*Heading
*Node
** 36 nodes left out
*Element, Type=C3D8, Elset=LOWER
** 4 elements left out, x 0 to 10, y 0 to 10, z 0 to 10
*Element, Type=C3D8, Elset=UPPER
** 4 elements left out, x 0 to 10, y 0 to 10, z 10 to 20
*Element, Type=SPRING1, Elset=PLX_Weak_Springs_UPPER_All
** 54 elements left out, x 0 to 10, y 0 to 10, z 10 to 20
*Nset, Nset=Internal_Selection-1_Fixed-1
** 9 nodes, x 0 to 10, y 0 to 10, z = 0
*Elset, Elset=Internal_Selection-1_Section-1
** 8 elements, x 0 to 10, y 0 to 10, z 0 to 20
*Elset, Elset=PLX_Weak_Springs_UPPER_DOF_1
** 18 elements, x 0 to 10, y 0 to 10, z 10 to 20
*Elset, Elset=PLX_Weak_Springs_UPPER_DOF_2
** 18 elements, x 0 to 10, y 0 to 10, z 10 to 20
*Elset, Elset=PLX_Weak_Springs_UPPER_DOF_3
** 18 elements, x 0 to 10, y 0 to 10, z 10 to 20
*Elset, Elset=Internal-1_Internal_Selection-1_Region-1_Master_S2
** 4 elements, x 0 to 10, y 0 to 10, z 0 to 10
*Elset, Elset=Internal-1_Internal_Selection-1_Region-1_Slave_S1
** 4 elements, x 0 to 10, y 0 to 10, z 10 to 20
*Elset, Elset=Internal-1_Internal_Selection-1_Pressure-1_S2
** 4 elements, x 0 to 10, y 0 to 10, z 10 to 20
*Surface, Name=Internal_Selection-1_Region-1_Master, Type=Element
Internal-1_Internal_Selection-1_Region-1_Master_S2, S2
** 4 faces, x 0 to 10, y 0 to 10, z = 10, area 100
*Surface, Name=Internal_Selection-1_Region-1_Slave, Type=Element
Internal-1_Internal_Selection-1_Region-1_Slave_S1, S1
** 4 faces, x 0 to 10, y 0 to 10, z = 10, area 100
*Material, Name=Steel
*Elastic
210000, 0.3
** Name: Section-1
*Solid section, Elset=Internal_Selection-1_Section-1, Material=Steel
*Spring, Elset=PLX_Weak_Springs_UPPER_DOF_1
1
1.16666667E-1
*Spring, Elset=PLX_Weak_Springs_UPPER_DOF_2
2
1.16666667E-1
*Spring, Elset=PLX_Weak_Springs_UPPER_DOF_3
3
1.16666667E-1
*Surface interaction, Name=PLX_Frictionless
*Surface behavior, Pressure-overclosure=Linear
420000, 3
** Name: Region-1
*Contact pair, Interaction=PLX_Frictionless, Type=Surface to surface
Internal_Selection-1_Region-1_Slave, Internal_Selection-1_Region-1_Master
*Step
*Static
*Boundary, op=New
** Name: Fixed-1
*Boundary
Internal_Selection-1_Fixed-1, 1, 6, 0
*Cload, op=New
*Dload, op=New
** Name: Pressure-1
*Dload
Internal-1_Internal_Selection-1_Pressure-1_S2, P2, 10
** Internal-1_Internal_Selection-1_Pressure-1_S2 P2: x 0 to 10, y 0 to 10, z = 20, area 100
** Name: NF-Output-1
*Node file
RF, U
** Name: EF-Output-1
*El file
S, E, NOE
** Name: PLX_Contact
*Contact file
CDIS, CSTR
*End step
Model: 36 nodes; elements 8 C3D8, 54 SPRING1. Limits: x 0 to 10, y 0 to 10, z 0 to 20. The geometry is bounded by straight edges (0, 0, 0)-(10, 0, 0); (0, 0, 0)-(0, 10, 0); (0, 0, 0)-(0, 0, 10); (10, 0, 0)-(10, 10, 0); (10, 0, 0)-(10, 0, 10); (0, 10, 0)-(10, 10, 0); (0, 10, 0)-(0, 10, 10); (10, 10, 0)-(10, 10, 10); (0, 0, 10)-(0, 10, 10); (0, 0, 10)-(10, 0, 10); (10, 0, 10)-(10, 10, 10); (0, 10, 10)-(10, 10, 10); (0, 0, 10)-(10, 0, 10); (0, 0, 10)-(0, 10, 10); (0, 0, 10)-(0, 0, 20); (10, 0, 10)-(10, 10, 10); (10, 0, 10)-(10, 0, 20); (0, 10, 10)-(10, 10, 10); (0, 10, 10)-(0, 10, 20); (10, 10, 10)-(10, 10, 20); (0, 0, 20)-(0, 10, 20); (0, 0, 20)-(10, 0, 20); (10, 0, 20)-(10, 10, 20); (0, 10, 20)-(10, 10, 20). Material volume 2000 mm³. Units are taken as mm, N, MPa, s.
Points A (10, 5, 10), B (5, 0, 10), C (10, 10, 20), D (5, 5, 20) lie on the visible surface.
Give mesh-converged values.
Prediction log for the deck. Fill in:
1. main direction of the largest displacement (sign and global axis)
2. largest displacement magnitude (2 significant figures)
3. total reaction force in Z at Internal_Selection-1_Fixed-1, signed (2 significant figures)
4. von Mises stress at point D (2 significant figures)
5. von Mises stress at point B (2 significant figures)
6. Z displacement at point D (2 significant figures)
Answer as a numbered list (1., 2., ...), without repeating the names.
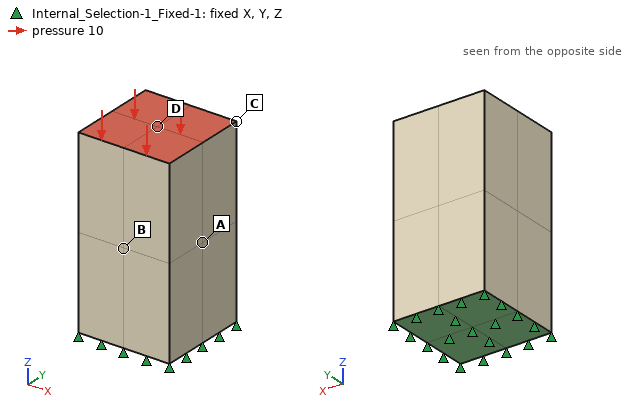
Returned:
1. -Z
2. 9.6e-04 mm
3. 1000 N
4. 10 MPa
5. 11 MPa
6. -9.5e-04 mm
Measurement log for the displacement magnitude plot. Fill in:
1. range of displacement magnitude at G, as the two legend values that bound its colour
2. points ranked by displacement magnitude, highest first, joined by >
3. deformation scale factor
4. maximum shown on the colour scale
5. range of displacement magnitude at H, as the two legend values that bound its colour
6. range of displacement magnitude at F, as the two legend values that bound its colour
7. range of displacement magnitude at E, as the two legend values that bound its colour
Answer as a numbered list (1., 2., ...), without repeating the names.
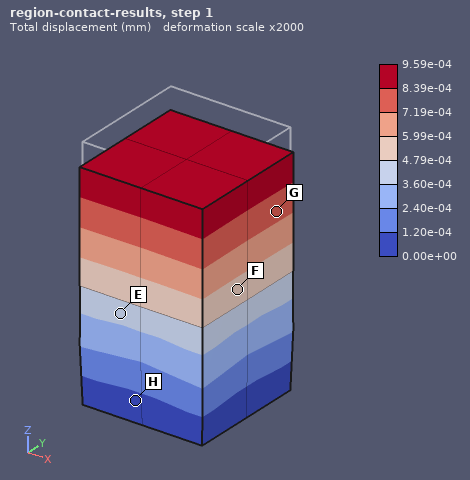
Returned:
1. 7.19e-04 to 8.39e-04 mm
2. G > F > E > H
3. 2000
4. 9.59e-04 mm
5. 0.00e+00 to 1.20e-04 mm
6. 4.79e-04 to 5.99e-04 mm
7. 3.60e-04 to 4.79e-04 mm
